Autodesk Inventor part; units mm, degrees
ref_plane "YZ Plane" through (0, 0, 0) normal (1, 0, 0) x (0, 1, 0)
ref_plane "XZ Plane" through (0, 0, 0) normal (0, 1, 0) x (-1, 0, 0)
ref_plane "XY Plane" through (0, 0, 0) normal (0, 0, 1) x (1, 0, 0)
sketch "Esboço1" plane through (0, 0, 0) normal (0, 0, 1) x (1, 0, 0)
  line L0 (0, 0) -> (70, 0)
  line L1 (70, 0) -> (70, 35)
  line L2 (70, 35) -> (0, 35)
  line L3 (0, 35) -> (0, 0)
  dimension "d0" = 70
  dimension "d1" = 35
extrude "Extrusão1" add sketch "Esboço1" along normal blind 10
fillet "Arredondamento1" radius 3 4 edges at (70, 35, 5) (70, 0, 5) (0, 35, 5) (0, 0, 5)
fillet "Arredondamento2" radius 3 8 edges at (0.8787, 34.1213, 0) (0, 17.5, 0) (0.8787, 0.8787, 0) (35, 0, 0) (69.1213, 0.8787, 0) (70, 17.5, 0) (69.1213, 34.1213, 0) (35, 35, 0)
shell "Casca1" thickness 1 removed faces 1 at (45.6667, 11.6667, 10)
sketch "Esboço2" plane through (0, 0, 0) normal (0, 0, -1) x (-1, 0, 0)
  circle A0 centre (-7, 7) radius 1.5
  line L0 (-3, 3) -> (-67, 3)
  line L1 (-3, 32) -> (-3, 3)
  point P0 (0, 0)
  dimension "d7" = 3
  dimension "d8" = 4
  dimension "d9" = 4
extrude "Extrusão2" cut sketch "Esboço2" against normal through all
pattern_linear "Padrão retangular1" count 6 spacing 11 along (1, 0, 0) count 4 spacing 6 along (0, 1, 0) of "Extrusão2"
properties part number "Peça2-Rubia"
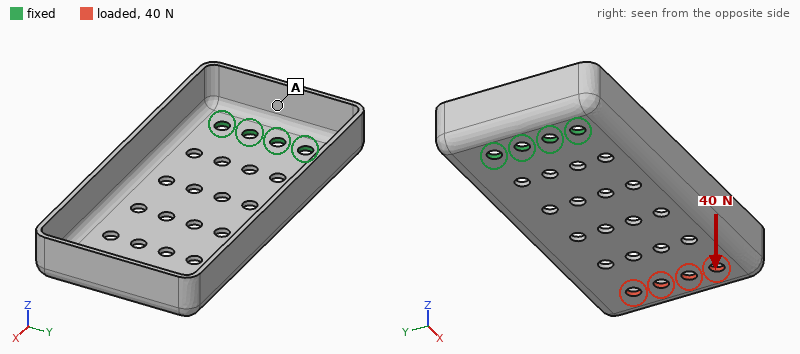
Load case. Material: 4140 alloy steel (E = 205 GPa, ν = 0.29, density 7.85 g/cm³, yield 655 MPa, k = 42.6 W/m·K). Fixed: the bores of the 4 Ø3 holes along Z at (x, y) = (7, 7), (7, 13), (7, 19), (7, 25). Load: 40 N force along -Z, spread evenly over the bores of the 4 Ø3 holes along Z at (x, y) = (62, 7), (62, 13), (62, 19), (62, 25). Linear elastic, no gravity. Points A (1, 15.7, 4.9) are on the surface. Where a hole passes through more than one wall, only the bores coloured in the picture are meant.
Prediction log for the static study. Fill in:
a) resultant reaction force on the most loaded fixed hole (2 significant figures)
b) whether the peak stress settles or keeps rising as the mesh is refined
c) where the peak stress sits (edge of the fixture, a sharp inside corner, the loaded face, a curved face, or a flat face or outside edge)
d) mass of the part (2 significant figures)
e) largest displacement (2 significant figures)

99 N
keeps rising
edge of the fixture
30 g
0.47 mm
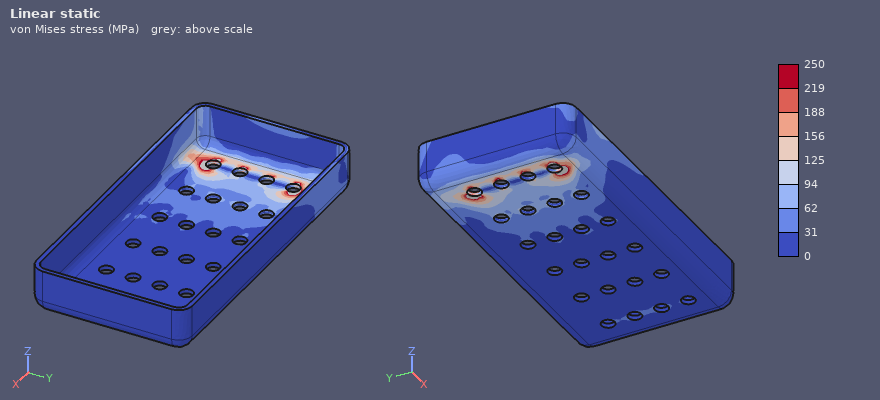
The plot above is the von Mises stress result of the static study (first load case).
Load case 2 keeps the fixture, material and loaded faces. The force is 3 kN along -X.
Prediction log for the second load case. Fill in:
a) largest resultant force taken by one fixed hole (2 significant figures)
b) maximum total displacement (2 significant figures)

1.0 kN
0.12 mm
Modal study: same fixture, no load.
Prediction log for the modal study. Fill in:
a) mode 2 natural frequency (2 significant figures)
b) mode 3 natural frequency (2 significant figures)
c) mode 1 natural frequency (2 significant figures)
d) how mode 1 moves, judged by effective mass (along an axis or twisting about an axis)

750 Hz
3200 Hz
440 Hz
along Z
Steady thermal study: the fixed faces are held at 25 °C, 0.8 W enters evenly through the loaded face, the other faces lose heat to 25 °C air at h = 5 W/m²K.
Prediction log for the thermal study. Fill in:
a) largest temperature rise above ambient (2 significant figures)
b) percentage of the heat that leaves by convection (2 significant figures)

18 K
41 %
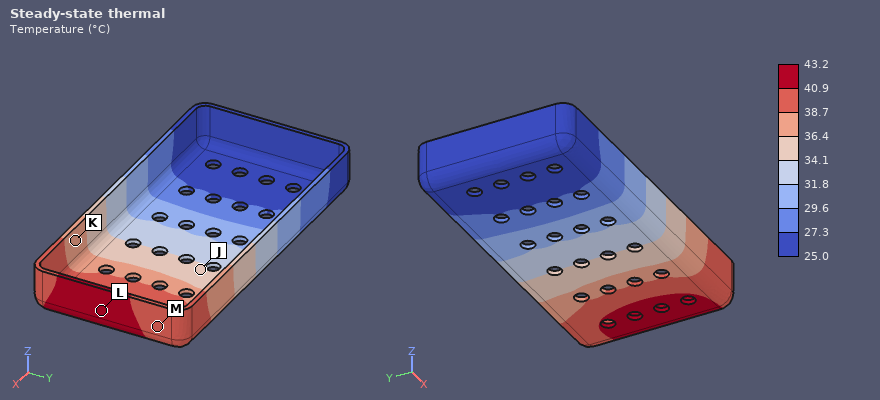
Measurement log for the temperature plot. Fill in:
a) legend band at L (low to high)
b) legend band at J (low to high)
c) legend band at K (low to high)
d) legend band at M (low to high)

40.9 to 43.2 °C
34.1 to 36.4 °C
36.4 to 38.7 °C
38.7 to 40.9 °C
